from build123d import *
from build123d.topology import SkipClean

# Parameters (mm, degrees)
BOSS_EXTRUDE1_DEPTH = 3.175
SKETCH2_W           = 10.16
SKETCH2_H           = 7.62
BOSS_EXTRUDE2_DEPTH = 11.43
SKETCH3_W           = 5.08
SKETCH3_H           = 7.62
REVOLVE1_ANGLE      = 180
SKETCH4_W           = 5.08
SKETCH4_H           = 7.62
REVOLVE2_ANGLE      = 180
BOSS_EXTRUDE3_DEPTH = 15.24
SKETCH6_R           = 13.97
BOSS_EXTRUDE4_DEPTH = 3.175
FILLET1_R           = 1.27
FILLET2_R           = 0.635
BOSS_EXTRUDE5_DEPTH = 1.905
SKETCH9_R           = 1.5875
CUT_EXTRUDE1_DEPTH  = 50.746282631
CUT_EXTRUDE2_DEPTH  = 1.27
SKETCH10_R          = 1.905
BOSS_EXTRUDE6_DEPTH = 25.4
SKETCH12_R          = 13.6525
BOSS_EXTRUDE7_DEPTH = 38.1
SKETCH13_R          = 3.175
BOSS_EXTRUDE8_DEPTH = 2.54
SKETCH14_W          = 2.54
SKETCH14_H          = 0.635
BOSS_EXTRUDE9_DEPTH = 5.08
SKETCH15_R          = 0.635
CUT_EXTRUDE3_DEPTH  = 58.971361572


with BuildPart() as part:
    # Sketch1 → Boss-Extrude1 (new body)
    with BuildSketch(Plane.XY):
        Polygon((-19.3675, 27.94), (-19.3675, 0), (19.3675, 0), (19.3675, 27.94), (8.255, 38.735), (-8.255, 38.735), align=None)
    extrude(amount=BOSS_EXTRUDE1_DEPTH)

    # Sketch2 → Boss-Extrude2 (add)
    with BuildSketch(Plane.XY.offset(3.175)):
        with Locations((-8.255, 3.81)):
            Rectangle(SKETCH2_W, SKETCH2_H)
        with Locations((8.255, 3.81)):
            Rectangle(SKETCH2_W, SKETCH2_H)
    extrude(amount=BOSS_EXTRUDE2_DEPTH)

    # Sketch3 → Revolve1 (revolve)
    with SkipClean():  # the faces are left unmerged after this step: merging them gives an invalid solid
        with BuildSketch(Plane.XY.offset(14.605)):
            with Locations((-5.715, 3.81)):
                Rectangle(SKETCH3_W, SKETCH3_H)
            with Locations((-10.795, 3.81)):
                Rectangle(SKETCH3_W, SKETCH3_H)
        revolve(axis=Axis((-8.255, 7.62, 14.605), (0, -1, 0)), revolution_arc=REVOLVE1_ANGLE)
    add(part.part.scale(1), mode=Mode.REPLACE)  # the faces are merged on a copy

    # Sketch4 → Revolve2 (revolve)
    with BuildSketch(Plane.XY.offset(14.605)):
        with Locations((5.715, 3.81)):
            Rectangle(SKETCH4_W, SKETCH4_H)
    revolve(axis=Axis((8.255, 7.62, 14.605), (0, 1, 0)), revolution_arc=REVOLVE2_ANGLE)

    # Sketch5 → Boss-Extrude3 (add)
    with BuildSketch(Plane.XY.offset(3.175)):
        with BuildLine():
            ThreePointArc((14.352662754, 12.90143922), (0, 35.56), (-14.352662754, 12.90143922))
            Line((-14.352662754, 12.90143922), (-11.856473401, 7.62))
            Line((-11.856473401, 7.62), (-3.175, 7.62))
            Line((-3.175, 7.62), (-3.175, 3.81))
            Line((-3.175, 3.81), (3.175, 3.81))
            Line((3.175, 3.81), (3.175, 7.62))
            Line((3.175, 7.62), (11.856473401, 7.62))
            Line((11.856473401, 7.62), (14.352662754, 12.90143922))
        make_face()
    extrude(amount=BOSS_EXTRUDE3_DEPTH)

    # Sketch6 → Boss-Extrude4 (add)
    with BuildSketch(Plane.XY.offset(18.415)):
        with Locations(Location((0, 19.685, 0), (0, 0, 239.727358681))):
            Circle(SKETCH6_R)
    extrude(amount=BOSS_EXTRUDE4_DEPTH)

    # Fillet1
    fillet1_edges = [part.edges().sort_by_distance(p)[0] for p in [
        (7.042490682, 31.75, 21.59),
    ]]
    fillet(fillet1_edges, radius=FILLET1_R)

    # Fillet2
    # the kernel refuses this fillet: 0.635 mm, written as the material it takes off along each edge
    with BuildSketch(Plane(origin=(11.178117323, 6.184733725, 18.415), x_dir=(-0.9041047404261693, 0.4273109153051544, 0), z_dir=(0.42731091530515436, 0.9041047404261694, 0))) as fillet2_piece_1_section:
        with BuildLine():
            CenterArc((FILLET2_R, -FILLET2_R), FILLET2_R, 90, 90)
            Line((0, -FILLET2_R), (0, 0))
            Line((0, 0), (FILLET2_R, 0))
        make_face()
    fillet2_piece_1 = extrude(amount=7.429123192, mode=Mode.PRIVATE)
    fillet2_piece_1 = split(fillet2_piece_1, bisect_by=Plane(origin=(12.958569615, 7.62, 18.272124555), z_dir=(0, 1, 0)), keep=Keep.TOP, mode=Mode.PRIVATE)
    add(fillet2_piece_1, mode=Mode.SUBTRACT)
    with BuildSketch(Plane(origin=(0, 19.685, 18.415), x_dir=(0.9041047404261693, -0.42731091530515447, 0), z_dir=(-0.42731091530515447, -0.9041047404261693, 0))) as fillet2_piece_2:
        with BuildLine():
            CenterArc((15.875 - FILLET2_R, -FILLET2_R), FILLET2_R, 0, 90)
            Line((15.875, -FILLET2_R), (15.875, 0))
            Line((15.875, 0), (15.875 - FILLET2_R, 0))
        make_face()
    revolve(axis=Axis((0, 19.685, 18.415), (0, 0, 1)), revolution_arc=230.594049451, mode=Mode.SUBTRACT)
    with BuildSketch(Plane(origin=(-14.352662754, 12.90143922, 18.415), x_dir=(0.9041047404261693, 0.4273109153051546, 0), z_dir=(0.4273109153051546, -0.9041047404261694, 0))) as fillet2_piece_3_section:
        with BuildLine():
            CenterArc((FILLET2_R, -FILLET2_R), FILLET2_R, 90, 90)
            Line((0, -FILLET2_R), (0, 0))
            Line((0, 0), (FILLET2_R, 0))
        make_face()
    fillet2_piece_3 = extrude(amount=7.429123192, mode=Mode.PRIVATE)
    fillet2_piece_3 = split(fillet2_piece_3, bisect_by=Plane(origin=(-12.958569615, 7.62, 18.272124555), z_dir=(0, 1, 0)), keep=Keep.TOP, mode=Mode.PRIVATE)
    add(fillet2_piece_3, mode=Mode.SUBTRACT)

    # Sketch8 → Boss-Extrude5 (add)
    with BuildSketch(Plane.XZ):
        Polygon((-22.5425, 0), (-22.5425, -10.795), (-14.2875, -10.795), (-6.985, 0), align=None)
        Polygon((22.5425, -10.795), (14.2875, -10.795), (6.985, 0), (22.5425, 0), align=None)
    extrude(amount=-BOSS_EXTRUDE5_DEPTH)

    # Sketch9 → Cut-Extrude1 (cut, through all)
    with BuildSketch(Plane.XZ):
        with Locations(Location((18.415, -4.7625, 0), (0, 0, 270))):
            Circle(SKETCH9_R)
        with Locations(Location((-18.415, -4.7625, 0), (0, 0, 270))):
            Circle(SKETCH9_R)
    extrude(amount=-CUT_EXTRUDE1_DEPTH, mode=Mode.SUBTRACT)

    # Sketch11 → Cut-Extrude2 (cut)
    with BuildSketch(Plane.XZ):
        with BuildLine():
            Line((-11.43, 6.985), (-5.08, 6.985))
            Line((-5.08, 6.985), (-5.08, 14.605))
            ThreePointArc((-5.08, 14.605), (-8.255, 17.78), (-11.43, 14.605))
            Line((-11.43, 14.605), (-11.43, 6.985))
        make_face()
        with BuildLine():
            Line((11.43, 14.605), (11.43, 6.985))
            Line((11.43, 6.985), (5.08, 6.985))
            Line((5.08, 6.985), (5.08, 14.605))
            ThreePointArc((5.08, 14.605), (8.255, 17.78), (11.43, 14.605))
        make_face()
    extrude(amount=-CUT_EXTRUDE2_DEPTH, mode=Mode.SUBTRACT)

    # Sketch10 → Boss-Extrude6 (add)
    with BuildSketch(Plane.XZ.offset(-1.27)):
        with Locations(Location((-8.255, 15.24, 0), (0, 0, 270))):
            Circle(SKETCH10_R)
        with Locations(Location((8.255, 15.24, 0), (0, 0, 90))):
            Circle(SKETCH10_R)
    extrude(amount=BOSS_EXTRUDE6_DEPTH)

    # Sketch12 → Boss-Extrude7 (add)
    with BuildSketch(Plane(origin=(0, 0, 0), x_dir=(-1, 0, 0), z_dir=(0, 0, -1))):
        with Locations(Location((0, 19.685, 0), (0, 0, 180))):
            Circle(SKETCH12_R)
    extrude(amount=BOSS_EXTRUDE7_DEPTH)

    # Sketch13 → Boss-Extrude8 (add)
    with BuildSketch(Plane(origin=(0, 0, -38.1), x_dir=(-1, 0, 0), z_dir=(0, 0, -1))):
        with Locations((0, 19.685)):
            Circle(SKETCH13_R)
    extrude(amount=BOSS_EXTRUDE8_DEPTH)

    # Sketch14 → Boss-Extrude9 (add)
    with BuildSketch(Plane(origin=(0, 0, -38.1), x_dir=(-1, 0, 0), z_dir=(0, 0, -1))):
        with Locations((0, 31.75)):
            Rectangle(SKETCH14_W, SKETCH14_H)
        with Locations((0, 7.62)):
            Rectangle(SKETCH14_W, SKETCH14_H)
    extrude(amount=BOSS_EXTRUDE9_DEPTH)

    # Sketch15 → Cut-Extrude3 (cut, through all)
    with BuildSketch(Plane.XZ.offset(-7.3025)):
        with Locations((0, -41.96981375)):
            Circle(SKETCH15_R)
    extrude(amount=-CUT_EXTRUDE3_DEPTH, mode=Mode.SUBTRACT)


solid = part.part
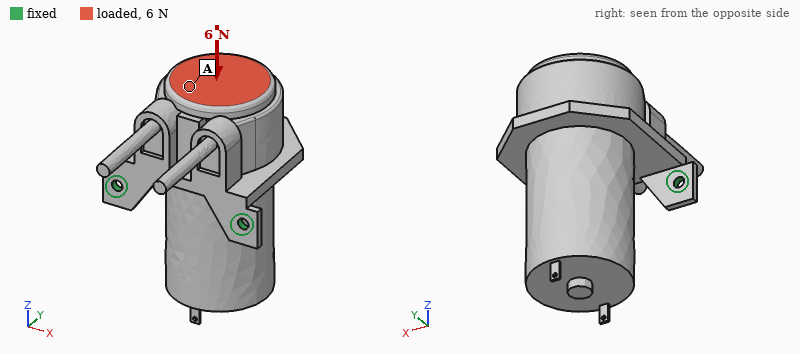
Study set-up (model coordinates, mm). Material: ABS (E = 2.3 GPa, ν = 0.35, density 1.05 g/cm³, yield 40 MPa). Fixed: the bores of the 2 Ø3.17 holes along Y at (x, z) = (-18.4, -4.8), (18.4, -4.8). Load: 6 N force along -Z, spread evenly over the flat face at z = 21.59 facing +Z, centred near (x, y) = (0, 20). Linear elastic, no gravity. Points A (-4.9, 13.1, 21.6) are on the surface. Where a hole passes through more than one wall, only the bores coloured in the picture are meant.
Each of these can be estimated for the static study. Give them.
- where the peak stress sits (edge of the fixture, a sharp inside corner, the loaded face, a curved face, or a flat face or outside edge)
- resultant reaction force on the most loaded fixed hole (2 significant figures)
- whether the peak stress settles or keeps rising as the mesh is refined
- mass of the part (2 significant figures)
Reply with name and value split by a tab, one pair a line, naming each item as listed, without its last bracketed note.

where the peak stress sits	edge of the fixture
resultant reaction force on the most loaded fixed hole	3.0 N
whether the peak stress settles or keeps rising as the mesh is refined	keeps rising
mass of the part	46 g
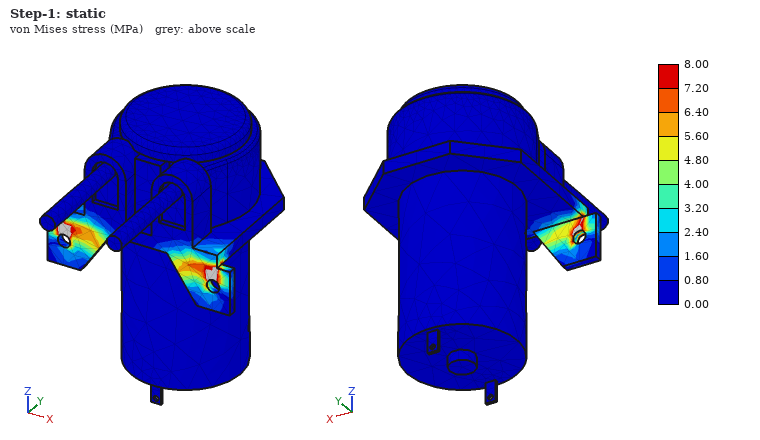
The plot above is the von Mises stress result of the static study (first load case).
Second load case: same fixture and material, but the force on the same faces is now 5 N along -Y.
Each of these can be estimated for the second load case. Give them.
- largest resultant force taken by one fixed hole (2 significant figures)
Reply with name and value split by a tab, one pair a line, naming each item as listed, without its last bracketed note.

largest resultant force taken by one fixed hole	3.3 N
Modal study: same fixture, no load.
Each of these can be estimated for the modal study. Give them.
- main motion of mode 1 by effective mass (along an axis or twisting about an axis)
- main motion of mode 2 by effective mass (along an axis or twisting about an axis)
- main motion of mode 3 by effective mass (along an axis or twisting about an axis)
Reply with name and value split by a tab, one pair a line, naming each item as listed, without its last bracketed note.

main motion of mode 1 by effective mass	along Z
main motion of mode 2 by effective mass	along X
main motion of mode 3 by effective mass	along Y
